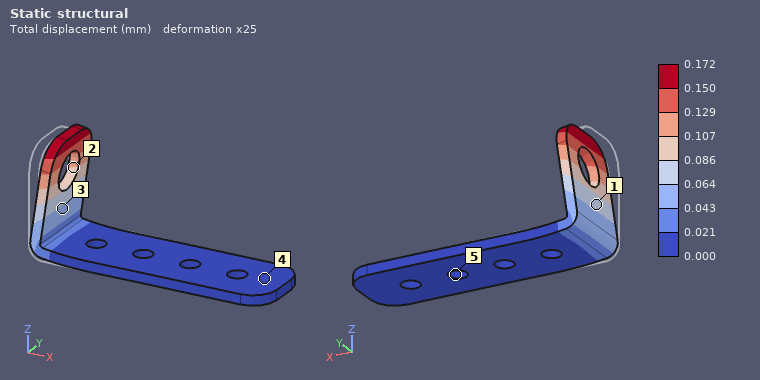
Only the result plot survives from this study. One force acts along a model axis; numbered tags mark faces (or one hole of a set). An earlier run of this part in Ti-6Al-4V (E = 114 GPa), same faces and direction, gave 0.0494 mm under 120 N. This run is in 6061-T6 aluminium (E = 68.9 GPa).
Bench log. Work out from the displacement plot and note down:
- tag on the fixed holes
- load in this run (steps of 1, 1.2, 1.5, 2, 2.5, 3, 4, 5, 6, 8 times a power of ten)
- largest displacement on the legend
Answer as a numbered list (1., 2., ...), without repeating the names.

1. 5
2. 250 N
3. 0.172 mm
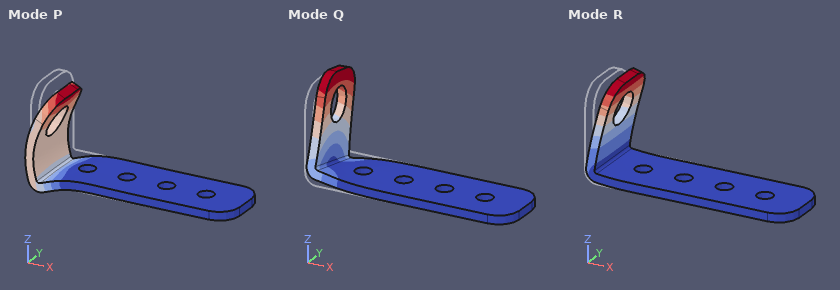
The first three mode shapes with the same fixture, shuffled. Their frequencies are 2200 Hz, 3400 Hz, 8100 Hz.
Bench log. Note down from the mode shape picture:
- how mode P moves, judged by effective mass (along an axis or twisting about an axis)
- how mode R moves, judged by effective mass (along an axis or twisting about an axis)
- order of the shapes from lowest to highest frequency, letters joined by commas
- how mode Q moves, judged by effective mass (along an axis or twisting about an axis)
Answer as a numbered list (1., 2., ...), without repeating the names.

1. along Z
2. along X
3. R, Q, P
4. along Y
